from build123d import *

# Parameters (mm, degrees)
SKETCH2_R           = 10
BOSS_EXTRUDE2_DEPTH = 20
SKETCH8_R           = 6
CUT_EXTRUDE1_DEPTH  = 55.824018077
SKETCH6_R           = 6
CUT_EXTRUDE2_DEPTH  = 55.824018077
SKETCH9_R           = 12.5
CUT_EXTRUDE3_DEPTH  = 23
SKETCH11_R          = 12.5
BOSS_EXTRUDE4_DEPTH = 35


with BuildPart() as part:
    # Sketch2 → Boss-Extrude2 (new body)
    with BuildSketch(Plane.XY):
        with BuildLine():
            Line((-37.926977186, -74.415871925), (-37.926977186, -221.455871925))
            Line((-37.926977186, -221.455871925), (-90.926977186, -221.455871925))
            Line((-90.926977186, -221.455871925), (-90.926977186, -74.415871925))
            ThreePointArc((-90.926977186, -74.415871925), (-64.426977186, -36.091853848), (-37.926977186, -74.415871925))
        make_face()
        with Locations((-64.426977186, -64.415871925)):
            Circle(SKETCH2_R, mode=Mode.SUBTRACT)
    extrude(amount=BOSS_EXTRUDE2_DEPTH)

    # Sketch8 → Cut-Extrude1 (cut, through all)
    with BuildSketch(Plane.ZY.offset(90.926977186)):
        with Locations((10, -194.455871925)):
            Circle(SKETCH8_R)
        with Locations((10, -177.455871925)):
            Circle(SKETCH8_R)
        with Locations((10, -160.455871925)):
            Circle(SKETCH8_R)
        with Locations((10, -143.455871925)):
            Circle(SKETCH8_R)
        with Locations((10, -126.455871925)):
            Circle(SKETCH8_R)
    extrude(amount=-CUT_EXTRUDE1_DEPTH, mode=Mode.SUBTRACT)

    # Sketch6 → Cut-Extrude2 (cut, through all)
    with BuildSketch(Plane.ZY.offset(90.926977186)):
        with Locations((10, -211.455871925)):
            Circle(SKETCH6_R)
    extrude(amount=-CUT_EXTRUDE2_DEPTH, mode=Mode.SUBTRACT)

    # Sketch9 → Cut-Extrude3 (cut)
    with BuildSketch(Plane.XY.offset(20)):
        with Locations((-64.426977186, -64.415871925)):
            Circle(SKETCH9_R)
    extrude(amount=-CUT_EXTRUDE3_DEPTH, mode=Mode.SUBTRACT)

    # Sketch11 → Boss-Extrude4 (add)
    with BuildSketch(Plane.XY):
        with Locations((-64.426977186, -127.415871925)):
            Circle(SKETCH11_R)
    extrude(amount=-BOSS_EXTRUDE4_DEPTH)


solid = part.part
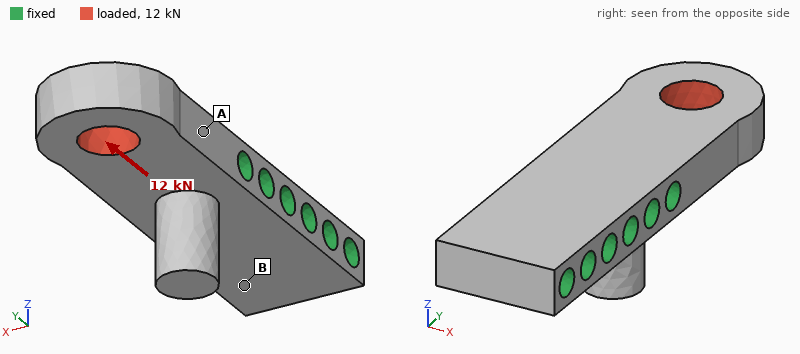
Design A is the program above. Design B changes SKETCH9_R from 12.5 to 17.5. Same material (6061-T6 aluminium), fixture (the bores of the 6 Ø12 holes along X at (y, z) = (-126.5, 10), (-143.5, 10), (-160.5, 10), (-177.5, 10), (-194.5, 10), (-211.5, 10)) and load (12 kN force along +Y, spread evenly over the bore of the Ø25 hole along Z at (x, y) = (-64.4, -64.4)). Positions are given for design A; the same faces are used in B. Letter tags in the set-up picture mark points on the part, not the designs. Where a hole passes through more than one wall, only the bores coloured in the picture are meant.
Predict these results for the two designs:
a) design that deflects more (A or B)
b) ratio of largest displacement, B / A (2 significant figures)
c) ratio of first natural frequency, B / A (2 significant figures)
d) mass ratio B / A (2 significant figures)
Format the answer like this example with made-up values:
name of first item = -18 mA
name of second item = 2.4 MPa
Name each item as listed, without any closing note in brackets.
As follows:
design that deflects more = B
ratio of largest displacement, B / A = 1.7
ratio of first natural frequency, B / A = 1.1
mass ratio B / A = 0.94
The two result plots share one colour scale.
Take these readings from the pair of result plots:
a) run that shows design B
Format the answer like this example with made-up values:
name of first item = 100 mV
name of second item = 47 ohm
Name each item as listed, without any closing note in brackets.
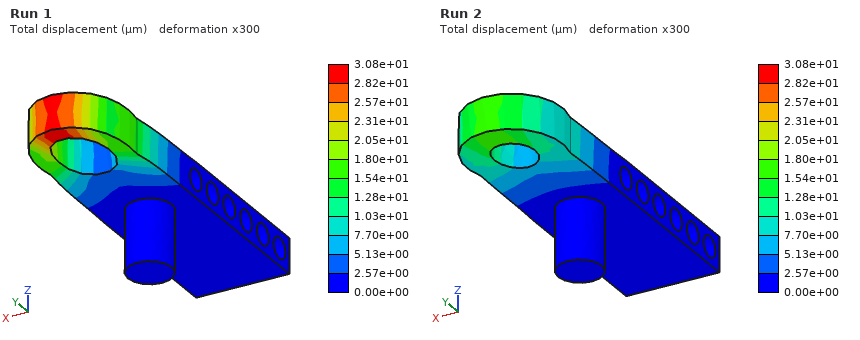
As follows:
run that shows design B = Run 1
